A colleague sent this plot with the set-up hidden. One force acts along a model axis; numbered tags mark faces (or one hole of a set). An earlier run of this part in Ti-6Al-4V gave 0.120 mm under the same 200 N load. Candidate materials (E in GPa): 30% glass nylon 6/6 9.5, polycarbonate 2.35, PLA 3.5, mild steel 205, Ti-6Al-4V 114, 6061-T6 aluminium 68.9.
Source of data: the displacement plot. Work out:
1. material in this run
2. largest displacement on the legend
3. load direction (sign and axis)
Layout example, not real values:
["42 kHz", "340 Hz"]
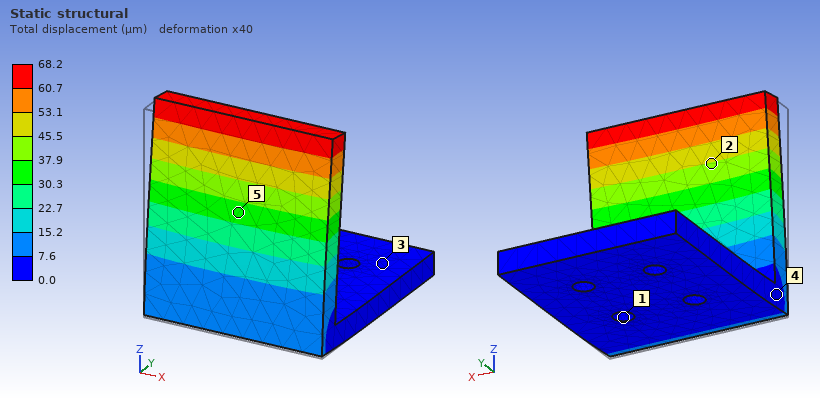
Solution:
["mild steel", "68.2 µm", "+Y"]
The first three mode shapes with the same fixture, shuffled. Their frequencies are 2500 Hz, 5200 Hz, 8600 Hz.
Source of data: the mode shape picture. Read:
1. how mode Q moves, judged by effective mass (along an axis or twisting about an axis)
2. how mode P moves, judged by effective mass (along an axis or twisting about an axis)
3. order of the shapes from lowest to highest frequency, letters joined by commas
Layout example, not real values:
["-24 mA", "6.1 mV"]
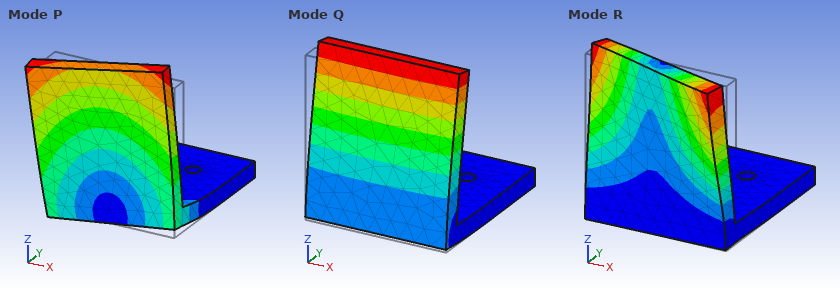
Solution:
["along Y", "along X", "Q, P, R"]
